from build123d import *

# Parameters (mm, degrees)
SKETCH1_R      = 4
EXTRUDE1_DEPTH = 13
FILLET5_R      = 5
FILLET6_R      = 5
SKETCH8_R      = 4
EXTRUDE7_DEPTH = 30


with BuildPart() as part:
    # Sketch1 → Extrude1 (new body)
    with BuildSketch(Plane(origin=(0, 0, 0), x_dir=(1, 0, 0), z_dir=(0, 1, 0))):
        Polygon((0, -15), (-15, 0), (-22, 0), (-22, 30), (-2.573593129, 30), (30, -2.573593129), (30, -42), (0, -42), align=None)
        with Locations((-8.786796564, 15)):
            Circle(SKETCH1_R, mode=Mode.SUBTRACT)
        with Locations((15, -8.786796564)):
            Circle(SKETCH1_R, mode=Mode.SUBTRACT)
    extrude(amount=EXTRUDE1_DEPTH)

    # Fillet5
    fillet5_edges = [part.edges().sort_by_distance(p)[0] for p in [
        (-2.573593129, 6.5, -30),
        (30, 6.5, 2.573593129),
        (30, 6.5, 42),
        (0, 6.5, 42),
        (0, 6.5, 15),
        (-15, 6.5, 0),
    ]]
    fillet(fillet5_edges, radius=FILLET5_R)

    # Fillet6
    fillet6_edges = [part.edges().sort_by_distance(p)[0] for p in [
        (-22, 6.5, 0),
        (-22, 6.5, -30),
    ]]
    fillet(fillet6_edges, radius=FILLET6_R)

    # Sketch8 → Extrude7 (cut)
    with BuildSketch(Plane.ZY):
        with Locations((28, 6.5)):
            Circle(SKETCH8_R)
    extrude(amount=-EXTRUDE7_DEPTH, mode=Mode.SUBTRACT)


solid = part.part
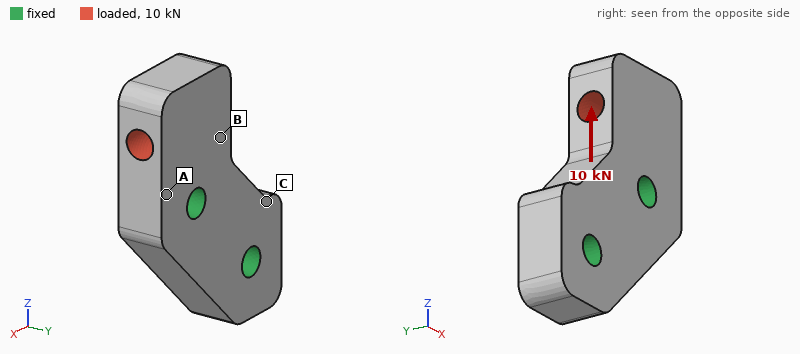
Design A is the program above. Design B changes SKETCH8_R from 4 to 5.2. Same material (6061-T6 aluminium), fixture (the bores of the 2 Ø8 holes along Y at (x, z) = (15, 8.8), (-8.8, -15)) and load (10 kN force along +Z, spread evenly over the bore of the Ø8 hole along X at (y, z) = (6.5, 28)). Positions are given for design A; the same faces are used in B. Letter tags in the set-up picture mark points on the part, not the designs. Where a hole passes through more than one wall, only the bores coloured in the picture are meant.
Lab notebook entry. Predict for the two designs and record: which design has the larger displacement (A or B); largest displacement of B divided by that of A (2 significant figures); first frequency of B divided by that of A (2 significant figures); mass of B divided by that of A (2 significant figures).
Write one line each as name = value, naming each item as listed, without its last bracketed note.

which design has the larger displacement = B
largest displacement of B divided by that of A = 1.4
first frequency of B divided by that of A = 0.81
mass of B divided by that of A = 0.96
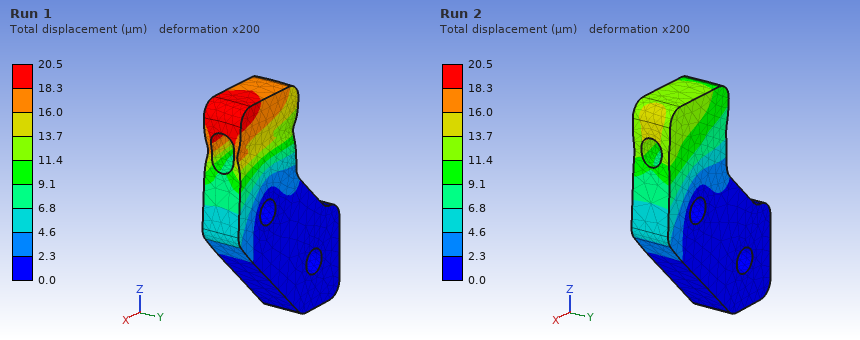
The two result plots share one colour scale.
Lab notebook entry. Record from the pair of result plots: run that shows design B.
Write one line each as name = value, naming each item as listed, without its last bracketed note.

run that shows design B = Run 1
